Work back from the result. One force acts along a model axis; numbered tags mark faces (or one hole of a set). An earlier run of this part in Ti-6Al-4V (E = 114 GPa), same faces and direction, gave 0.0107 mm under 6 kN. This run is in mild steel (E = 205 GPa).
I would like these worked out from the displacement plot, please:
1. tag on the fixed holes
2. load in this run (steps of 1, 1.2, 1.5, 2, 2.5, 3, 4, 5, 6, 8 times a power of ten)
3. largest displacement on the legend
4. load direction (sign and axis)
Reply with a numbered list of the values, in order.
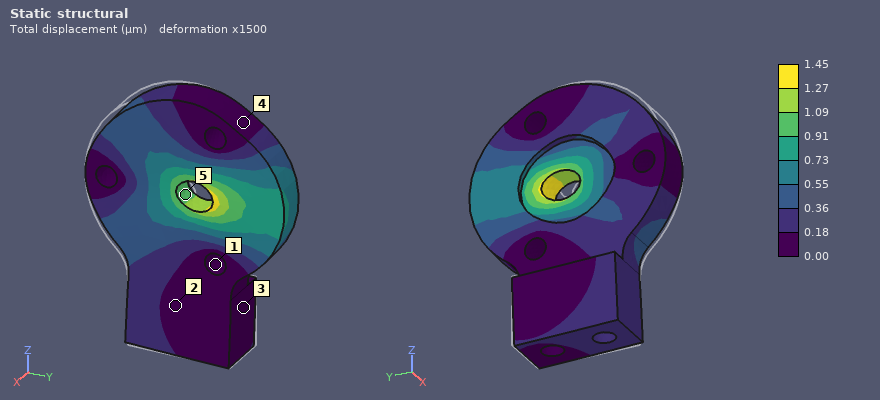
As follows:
1. 1
2. 1.5 kN
3. 1.45 µm
4. +Y
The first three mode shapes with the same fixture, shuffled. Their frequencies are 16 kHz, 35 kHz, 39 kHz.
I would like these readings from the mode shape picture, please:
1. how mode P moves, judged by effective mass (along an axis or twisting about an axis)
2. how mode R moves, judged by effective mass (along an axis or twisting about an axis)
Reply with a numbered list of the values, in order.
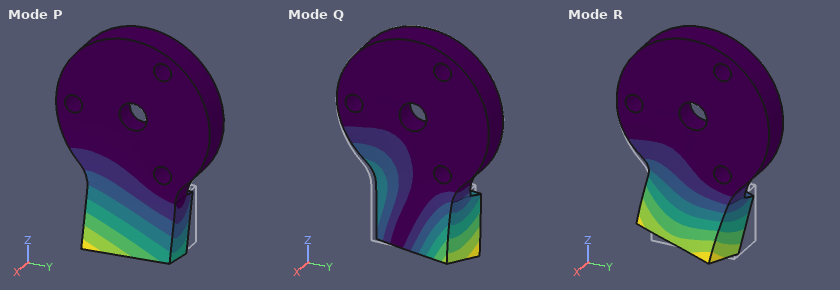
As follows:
1. along X
2. along Y
